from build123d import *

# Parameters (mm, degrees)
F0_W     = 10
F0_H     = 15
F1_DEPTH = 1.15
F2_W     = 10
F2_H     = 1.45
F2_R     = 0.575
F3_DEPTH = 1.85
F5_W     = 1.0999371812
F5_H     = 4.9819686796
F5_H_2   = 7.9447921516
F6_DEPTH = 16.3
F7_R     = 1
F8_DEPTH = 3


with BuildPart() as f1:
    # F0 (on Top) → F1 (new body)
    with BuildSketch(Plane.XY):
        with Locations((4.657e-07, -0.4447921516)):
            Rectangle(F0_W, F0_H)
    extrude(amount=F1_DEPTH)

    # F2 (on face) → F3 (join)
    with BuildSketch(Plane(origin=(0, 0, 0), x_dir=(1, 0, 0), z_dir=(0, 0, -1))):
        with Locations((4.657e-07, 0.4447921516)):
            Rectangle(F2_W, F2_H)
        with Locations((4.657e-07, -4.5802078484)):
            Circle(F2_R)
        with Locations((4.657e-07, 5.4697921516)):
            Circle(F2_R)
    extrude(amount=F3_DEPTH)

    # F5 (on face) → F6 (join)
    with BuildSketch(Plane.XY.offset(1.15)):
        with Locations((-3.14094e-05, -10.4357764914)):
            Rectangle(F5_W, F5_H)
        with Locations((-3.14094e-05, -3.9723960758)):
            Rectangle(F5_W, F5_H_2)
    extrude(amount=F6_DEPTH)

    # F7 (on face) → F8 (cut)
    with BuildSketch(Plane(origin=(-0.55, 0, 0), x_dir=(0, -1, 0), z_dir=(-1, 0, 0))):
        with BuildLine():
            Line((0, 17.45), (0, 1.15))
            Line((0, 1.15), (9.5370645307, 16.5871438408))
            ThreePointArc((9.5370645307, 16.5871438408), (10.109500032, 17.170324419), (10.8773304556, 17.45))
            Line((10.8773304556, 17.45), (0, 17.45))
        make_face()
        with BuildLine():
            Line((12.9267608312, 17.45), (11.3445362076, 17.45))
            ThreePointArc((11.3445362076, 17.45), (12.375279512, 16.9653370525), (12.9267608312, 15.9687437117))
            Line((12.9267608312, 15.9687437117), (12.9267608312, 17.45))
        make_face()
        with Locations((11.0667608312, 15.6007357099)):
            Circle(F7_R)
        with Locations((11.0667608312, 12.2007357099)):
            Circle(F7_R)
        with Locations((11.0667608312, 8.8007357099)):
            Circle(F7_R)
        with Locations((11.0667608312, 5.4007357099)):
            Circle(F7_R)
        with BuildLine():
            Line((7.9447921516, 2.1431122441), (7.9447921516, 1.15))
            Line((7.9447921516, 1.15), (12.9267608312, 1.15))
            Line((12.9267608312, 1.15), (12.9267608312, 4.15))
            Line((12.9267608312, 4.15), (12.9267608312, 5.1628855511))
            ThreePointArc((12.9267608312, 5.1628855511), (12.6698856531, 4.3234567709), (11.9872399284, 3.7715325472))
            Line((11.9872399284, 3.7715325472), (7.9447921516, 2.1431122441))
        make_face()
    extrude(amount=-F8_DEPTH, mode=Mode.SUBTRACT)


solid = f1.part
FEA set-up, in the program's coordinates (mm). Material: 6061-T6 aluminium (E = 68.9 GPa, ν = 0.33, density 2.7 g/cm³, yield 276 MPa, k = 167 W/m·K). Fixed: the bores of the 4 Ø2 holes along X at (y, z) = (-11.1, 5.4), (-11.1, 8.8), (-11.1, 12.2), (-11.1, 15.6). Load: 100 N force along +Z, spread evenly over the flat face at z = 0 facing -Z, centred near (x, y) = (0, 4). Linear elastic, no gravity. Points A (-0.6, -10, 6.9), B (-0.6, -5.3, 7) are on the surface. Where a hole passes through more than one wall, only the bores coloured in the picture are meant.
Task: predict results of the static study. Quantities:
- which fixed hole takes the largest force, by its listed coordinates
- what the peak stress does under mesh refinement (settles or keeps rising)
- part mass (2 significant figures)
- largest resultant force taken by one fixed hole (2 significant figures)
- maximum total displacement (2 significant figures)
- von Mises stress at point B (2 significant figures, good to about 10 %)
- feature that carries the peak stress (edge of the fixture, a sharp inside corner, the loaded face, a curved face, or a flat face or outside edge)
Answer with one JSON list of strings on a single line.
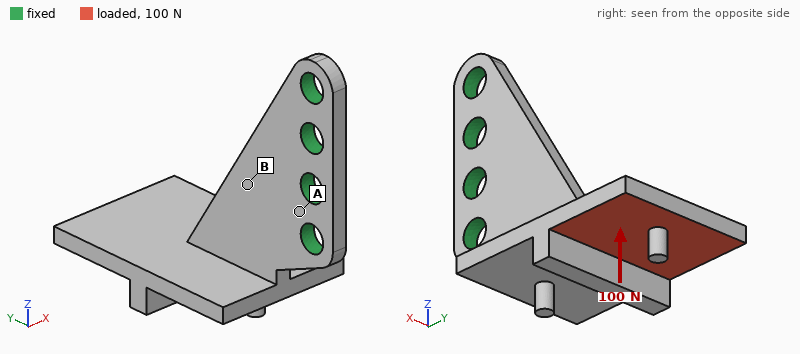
["(-11.1, 5.4)", "keeps rising", "0.86 g", "210 N", "0.17 mm", "72 MPa", "a sharp inside corner"]
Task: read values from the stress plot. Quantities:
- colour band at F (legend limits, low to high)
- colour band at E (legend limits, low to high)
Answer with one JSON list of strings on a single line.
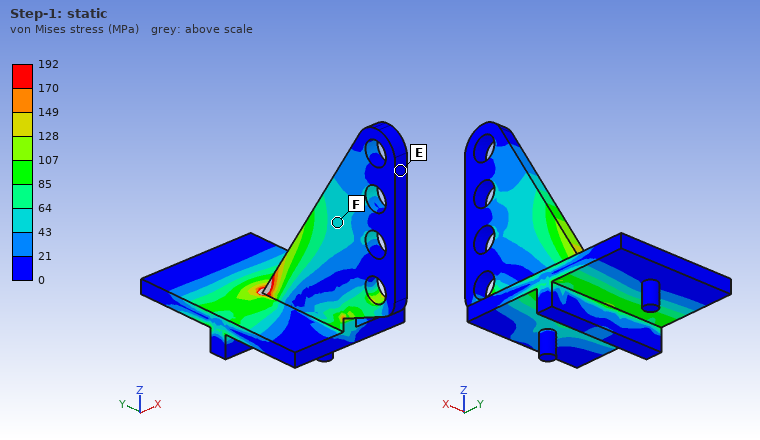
["43 to 64 MPa", "0 to 21 MPa"]
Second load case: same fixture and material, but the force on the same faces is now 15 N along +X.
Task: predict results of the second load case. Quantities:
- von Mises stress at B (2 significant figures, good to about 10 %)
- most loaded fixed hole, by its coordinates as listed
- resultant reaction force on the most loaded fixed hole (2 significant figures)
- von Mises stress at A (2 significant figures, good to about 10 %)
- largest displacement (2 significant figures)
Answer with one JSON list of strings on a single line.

["99 MPa", "(-11.1, 5.4)", "25 N", "77 MPa", "0.34 mm"]
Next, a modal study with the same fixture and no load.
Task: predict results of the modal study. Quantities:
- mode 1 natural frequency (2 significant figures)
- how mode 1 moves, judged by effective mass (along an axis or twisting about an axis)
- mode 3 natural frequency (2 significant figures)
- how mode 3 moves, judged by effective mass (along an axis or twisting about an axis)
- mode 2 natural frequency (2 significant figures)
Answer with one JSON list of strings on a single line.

["2100 Hz", "along X", "9200 Hz", "along Z", "6500 Hz"]
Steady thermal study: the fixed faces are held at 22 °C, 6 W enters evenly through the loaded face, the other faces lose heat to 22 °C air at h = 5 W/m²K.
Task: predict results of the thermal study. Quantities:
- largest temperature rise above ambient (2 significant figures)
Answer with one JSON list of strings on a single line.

["60 K"]
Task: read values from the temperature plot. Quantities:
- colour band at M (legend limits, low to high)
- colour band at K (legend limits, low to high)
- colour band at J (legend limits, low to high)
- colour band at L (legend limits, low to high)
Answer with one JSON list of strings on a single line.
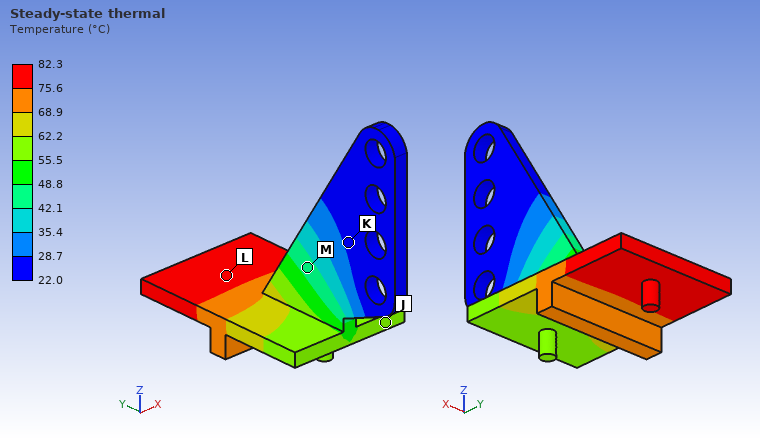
["42.1 to 48.8 °C", "22.0 to 28.7 °C", "55.5 to 62.2 °C", "75.6 to 82.3 °C"]
